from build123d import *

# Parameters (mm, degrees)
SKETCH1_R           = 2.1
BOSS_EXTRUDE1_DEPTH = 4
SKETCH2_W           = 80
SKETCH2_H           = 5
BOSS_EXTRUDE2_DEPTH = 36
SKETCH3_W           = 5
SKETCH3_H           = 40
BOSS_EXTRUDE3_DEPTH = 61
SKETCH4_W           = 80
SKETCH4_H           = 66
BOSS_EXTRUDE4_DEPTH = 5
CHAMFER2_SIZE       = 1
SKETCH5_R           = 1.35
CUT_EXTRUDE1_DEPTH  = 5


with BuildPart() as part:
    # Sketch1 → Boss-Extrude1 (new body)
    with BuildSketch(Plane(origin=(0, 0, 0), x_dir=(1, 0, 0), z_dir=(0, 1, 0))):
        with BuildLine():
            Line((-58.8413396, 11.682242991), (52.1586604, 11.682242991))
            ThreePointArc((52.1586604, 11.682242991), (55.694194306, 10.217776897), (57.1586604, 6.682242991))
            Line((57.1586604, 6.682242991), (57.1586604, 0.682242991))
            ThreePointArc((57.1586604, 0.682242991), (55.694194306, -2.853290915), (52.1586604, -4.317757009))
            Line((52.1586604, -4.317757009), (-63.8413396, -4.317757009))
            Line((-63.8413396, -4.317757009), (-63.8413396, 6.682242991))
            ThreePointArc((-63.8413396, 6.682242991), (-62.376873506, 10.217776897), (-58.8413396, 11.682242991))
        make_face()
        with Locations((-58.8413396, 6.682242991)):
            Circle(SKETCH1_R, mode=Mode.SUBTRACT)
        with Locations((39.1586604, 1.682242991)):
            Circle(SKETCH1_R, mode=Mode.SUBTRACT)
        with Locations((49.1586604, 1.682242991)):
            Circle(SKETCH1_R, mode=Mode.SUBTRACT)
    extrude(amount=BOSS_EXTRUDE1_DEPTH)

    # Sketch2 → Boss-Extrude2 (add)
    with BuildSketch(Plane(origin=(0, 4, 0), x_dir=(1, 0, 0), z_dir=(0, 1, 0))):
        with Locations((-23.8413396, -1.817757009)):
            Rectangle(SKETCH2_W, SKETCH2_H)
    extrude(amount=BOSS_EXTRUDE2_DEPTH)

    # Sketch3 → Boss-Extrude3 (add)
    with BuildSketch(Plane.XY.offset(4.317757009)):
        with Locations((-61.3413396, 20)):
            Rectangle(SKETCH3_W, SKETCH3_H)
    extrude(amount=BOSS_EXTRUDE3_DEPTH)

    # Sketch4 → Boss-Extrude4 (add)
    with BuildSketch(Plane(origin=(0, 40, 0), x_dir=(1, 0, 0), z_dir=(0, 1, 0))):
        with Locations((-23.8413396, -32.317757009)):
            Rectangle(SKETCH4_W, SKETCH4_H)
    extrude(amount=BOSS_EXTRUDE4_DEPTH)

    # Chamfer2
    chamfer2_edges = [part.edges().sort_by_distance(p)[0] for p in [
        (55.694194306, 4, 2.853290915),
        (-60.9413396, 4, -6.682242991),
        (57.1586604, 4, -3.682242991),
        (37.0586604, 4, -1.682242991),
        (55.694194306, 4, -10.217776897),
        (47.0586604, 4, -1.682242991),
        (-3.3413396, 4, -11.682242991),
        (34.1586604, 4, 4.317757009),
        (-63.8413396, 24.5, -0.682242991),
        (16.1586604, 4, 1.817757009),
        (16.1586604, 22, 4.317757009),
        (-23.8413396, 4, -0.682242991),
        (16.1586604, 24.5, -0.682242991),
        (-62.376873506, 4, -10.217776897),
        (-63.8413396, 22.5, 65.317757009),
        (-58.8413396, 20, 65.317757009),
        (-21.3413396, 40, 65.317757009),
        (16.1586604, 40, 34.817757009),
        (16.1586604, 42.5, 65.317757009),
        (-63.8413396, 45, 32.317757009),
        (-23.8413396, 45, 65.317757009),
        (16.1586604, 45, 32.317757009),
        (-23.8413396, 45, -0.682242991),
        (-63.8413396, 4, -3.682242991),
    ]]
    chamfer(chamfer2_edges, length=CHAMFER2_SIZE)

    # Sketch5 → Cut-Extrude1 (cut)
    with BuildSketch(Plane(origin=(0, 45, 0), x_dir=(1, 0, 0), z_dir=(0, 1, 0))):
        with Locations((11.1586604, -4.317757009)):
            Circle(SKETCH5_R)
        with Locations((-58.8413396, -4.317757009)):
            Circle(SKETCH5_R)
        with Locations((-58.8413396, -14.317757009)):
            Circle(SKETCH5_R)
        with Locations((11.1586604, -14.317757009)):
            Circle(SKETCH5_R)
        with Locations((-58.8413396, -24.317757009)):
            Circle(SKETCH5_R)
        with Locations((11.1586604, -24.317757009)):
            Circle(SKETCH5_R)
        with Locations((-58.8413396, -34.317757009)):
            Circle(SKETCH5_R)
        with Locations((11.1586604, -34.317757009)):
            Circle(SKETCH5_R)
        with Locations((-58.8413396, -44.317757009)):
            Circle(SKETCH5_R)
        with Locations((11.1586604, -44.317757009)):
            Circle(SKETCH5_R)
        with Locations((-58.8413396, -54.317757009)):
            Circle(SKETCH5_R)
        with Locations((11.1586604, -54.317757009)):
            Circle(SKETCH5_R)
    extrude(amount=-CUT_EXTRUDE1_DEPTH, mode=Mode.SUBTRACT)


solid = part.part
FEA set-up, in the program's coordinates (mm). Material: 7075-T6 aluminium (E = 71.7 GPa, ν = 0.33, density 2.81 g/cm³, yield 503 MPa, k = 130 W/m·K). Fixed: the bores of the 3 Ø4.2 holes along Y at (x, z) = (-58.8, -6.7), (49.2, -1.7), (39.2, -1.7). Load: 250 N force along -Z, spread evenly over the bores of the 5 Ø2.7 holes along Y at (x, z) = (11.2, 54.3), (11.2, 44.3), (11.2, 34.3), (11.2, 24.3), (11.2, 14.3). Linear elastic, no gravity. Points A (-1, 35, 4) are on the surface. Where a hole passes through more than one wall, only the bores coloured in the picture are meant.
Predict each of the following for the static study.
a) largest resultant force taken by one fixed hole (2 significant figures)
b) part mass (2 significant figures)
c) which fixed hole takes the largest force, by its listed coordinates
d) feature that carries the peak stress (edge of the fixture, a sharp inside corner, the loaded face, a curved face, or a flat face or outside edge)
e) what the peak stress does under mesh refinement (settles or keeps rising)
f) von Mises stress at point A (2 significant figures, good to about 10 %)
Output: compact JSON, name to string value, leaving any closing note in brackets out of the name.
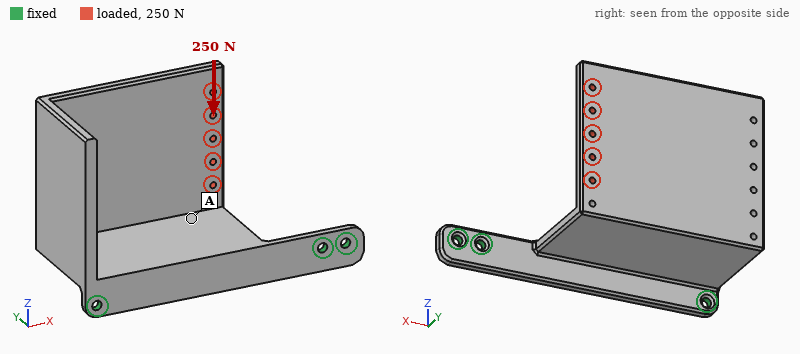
{"largest resultant force taken by one fixed hole": "340 N", "part mass": "170 g", "which fixed hole takes the largest force, by its listed coordinates": "(39.2, -1.7)", "feature that carries the peak stress": "edge of the fixture", "what the peak stress does under mesh refinement": "keeps rising", "von Mises stress at point A": "17 MPa"}
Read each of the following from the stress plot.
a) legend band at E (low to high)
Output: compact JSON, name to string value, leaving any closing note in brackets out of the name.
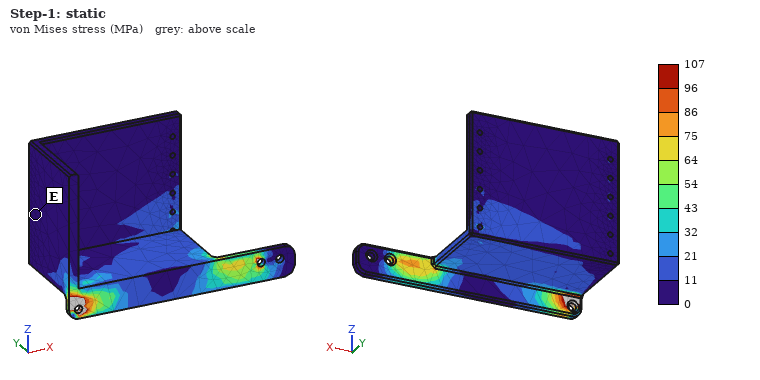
{"legend band at E": "0 to 11 MPa"}
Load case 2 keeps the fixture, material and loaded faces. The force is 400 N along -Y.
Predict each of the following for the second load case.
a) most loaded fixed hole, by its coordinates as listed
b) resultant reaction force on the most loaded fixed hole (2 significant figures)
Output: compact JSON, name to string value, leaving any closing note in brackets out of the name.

{"most loaded fixed hole, by its coordinates as listed": "(39.2, -1.7)", "resultant reaction force on the most loaded fixed hole": "450 N"}
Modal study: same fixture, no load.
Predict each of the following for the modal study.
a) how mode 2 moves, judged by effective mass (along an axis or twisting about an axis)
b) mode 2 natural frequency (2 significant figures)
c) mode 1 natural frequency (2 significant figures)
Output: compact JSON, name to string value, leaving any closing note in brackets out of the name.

{"how mode 2 moves, judged by effective mass": "along X", "mode 2 natural frequency": "750 Hz", "mode 1 natural frequency": "280 Hz"}
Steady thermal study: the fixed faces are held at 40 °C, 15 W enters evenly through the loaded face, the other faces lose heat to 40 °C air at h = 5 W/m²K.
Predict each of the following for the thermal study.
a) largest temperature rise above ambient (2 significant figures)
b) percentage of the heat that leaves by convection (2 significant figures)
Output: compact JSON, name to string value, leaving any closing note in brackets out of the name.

{"largest temperature rise above ambient": "35 K", "percentage of the heat that leaves by convection": "16 %"}
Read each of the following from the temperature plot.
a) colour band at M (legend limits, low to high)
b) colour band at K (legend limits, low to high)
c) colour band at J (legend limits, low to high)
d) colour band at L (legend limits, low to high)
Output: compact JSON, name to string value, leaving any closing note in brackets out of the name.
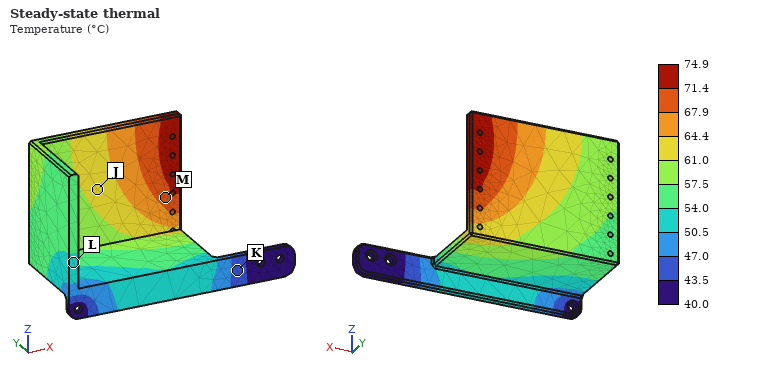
{"colour band at M": "67.9 to 71.4 °C", "colour band at K": "43.5 to 47.0 °C", "colour band at J": "61.0 to 64.4 °C", "colour band at L": "50.5 to 54.0 °C"}
